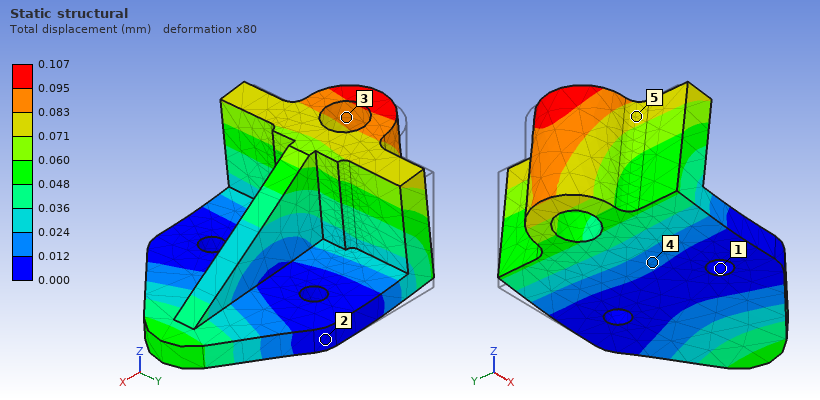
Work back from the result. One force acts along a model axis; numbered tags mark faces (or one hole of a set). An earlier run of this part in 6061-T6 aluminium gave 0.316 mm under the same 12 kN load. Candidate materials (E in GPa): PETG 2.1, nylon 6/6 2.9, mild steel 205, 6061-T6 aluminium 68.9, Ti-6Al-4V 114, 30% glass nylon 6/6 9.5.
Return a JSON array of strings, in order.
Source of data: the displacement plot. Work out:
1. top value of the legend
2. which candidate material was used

["0.107 mm", "mild steel"]
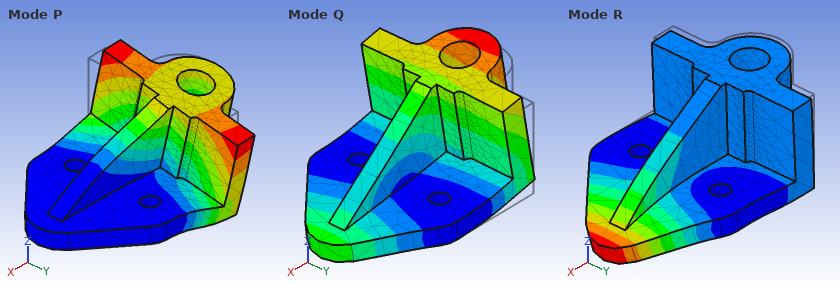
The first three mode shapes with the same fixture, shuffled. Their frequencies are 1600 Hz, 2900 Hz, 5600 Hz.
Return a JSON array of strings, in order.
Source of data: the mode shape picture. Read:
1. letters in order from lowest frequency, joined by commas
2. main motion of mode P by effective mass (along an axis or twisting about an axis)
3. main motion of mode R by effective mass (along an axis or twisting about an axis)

["Q, P, R", "along Y", "along Z"]
